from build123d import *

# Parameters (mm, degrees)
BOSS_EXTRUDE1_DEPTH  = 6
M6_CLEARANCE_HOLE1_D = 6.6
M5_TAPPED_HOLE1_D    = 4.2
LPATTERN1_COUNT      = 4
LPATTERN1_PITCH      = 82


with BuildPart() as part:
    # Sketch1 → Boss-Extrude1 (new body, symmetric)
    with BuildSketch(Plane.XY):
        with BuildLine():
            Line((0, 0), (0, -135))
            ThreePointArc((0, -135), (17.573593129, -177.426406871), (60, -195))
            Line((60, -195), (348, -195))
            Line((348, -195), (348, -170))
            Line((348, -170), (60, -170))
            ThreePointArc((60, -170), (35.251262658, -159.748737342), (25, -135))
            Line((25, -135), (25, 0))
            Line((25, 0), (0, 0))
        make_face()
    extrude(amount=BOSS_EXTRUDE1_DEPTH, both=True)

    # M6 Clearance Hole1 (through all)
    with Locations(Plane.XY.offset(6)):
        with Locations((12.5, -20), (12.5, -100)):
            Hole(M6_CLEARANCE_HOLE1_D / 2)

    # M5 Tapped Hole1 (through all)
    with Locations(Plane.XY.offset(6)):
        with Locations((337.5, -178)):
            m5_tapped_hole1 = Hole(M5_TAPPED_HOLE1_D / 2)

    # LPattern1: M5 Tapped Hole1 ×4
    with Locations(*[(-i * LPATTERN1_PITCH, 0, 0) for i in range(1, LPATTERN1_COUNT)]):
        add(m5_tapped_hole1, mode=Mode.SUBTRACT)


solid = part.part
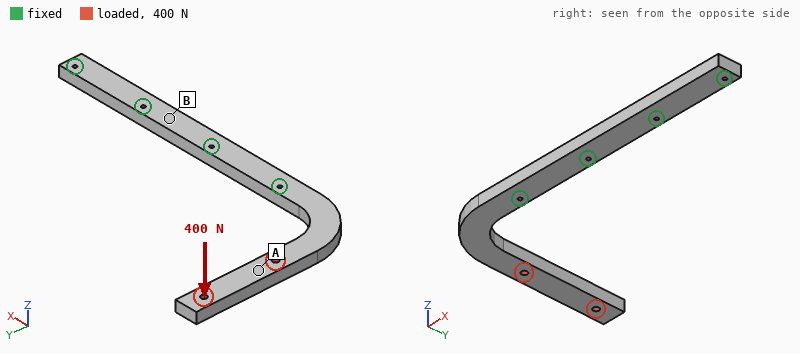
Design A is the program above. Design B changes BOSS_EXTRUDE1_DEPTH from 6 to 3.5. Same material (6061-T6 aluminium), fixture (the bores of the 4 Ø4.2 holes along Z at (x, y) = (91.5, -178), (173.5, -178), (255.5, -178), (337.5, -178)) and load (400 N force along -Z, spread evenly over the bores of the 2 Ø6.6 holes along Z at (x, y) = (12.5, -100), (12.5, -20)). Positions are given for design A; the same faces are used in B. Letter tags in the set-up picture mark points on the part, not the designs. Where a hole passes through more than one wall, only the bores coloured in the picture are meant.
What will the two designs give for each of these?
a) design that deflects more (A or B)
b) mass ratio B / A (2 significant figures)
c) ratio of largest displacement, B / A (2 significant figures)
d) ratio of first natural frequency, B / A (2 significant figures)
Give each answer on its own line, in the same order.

B
0.58
4.6
0.61
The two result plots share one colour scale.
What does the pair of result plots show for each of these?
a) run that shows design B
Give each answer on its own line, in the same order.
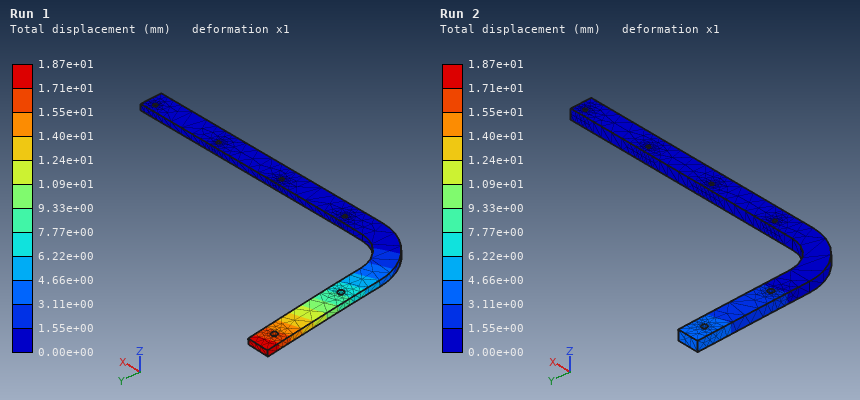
Run 1
